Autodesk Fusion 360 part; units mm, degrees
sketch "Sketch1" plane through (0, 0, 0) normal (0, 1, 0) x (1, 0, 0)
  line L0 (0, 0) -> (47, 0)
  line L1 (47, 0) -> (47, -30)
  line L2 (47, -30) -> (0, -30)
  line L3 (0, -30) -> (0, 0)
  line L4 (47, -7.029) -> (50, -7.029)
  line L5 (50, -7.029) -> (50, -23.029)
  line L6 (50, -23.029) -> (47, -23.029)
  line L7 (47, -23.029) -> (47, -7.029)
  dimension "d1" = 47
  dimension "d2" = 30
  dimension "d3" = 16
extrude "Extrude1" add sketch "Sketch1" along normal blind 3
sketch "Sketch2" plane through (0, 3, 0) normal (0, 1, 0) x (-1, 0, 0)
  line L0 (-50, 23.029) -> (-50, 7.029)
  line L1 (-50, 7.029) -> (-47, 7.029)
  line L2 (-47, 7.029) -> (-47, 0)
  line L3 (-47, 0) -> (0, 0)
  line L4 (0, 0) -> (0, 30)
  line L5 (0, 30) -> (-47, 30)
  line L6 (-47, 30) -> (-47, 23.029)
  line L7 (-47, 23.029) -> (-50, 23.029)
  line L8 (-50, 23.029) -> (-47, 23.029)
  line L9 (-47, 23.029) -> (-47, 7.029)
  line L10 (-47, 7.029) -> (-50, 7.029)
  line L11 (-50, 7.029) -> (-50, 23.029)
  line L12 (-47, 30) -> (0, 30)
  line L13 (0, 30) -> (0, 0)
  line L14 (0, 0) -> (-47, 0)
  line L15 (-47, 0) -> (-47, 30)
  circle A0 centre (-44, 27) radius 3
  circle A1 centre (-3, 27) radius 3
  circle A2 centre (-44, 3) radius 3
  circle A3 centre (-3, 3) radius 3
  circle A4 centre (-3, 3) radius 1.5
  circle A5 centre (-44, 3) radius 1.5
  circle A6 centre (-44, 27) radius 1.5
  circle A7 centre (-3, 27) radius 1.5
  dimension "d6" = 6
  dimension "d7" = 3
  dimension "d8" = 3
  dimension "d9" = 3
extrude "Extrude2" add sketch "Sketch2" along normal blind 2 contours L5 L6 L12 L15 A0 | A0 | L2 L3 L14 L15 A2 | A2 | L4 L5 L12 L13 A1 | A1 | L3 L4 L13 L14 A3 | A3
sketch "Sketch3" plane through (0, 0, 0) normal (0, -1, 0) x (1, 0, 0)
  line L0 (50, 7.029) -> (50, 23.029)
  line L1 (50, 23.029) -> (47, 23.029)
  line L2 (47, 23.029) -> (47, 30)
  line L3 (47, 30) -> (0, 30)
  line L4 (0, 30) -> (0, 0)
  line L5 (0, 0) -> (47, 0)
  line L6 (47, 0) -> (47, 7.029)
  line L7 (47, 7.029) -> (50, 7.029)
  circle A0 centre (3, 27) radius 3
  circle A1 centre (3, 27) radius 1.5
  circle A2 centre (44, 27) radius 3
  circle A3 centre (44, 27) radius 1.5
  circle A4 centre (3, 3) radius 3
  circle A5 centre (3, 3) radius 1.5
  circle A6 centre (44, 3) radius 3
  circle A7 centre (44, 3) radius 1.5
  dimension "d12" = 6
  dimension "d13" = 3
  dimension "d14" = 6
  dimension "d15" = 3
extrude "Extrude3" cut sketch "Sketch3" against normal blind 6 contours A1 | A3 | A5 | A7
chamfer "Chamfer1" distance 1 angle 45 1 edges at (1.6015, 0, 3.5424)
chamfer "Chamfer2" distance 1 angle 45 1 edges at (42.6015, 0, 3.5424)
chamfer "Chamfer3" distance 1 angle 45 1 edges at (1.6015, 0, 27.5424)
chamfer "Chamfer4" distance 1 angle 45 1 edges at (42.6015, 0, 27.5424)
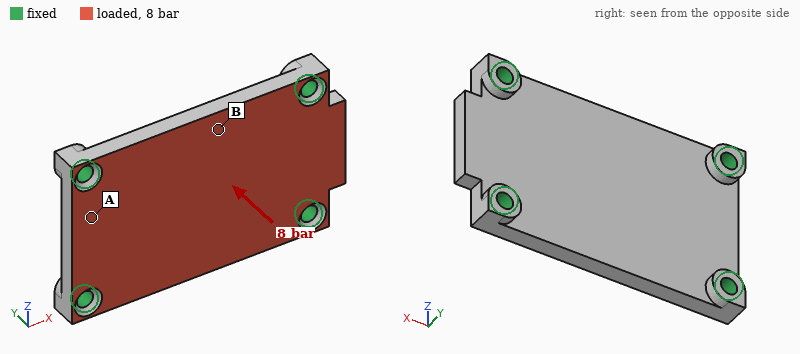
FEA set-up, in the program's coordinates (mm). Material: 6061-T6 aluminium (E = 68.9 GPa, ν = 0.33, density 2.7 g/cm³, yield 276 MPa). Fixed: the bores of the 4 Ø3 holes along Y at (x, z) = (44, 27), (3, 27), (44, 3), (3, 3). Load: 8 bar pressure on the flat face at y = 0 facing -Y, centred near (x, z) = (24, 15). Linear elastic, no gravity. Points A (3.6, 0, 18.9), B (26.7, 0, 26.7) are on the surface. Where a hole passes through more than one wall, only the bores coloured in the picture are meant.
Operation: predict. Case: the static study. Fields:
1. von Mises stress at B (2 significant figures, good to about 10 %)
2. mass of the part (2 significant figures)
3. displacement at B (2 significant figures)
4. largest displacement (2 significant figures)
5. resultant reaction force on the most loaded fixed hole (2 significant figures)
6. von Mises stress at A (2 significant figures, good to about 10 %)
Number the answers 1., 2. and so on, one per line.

1. 40 MPa
2. 12 g
3. 42 µm
4. 46 µm
5. 320 N
6. 19 MPa
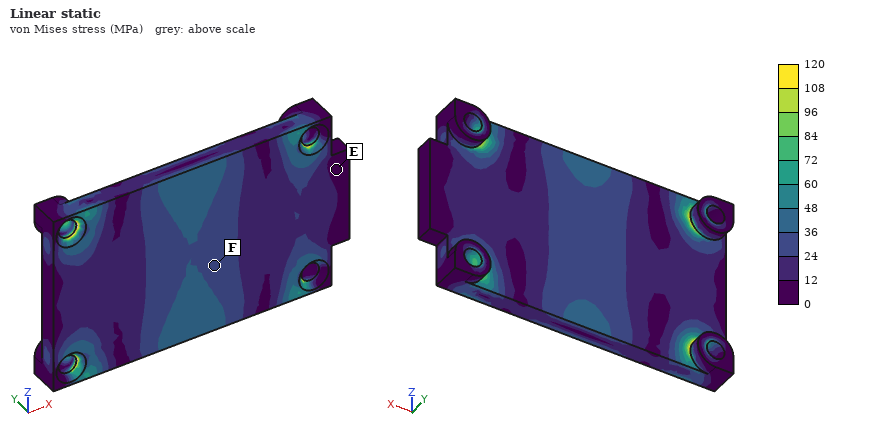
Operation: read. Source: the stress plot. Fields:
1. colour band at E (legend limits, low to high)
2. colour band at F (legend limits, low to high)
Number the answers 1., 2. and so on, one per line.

1. 0 to 12 MPa
2. 24 to 36 MPa
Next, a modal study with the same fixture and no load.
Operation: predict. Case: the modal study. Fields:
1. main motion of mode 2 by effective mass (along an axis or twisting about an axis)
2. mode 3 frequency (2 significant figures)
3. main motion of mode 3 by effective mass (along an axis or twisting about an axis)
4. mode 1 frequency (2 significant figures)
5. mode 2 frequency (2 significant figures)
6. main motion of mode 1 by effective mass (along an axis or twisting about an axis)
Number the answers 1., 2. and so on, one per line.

1. twisting about X
2. 21 kHz
3. twisting about Z
4. 8400 Hz
5. 13 kHz
6. along Y
